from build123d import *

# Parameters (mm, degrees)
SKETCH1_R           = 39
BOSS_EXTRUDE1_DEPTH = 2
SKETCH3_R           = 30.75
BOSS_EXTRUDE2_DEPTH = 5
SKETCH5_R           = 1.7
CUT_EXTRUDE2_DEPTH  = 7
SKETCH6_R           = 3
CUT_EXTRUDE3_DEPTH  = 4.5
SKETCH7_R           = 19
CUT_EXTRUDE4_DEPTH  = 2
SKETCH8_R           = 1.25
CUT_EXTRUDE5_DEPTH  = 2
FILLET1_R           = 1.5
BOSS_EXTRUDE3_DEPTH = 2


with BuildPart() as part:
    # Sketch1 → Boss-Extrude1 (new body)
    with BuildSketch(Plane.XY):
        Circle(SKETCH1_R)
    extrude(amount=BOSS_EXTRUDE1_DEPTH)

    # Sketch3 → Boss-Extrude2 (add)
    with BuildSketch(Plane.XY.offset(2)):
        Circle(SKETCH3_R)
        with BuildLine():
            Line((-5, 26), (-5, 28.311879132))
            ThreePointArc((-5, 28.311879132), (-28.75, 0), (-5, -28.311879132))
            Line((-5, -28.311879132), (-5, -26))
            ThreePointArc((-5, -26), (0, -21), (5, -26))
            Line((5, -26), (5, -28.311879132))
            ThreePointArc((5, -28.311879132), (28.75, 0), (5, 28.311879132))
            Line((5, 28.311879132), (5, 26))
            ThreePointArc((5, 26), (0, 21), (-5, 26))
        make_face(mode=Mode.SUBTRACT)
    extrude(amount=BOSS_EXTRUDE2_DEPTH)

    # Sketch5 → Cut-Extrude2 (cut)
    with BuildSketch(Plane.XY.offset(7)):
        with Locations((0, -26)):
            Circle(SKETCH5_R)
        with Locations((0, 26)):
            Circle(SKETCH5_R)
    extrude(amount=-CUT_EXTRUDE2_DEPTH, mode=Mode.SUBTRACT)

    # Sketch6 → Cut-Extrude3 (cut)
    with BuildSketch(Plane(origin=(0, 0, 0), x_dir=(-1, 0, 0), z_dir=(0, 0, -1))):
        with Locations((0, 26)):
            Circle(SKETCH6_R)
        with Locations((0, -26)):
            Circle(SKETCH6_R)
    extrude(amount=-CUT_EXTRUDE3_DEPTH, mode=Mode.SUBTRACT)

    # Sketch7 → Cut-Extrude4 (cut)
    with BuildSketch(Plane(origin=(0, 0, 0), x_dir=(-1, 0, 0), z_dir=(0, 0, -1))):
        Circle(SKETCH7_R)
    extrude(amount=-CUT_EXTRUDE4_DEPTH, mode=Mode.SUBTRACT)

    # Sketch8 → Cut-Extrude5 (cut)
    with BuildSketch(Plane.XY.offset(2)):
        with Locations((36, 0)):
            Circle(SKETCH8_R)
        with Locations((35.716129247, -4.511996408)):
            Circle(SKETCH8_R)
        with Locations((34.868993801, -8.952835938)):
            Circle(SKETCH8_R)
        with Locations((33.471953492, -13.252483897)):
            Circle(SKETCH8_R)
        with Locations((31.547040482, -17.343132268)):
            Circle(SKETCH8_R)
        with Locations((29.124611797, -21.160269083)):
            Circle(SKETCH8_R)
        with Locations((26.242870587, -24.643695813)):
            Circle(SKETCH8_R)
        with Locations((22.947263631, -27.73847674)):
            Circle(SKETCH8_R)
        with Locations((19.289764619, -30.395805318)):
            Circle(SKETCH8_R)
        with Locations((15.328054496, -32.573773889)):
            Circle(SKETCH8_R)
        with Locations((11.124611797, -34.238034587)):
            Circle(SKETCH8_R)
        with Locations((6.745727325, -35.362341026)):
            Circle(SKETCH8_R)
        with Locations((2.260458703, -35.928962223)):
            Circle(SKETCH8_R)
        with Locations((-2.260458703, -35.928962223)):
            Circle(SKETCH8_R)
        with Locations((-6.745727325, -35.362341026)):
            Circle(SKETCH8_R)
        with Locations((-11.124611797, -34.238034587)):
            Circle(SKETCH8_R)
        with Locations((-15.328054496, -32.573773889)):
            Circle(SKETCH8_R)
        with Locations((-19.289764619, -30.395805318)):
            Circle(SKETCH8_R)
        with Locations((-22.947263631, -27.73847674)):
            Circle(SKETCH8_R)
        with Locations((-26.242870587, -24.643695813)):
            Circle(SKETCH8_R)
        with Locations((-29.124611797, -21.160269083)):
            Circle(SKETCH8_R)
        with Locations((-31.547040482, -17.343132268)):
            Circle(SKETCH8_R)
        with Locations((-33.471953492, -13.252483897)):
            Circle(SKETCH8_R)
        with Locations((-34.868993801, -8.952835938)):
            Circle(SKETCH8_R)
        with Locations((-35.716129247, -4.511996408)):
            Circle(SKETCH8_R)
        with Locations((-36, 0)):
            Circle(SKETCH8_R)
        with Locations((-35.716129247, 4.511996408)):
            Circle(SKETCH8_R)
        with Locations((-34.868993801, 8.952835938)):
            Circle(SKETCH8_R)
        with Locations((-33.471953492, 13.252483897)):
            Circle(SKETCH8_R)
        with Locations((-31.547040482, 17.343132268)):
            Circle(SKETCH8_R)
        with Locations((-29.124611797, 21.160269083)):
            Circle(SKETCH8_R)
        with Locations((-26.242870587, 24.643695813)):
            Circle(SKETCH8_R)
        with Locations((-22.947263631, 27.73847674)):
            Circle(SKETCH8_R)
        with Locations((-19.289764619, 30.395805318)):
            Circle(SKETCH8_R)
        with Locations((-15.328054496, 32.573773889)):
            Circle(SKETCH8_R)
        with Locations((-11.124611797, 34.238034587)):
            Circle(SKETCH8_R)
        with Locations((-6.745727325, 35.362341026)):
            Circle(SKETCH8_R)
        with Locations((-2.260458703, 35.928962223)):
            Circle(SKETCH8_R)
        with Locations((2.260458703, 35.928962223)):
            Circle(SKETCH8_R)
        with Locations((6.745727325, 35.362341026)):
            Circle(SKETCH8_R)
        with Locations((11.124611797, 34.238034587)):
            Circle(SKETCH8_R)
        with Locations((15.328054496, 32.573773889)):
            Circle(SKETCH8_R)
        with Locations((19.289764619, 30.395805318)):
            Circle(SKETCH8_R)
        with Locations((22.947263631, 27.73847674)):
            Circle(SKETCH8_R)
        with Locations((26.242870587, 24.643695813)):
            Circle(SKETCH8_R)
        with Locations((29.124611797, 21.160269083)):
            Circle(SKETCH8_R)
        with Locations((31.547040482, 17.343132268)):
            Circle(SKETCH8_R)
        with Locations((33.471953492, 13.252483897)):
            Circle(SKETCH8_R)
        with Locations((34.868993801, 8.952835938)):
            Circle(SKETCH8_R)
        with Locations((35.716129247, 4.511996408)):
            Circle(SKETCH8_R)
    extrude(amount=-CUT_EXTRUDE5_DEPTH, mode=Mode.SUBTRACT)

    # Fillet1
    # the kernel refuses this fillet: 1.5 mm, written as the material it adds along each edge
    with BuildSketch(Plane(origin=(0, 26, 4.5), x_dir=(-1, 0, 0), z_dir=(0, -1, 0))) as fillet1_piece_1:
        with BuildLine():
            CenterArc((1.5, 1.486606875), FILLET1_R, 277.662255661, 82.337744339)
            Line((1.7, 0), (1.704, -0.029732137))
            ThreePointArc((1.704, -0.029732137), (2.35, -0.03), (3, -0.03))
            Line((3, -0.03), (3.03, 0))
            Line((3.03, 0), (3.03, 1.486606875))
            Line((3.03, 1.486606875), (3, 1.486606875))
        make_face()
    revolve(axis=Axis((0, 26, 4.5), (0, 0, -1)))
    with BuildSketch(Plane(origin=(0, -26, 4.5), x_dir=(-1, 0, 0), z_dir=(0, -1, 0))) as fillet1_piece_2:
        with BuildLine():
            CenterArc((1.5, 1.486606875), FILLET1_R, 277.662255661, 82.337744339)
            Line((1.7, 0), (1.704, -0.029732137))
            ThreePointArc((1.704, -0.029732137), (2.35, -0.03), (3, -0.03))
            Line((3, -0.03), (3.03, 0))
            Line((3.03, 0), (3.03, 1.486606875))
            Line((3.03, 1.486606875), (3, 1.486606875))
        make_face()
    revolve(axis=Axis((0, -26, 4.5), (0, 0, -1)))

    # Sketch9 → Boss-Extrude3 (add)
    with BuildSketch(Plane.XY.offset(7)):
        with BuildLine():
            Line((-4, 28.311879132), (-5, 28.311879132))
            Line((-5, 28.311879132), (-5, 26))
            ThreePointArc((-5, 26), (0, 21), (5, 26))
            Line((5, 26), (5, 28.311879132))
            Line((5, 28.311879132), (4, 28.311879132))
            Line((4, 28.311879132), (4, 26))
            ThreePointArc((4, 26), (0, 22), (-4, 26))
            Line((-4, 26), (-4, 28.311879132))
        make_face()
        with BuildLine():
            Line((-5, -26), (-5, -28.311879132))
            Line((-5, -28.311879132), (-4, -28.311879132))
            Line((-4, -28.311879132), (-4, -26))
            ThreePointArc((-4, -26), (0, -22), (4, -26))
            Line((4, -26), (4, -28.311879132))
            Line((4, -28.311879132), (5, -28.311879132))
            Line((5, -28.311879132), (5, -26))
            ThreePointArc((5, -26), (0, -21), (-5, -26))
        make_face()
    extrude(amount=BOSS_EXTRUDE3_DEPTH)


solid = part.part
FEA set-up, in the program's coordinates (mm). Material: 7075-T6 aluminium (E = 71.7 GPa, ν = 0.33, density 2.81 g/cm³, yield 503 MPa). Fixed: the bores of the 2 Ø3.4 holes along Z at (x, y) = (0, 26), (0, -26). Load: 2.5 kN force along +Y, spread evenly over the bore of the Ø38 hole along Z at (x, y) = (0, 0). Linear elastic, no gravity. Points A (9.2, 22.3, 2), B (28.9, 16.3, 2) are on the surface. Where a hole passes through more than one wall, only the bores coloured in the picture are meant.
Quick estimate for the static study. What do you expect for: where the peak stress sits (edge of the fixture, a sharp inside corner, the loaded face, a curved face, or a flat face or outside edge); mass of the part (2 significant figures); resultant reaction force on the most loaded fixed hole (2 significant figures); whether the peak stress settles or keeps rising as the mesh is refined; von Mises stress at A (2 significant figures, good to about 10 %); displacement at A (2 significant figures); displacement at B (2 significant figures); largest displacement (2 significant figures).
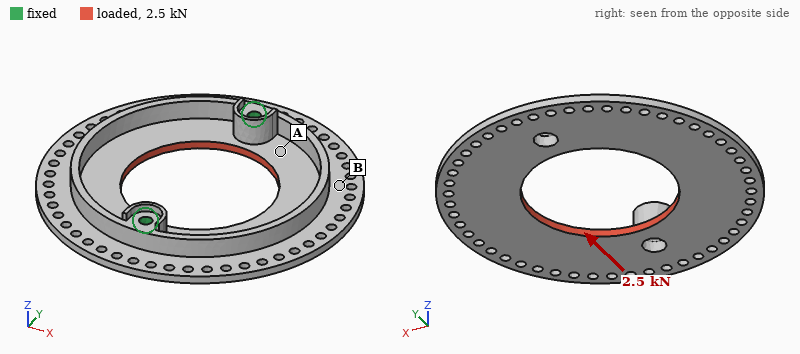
edge of the fixture
26 g
1.3 kN
keeps rising
42 MPa
21 µm
28 µm
42 µm
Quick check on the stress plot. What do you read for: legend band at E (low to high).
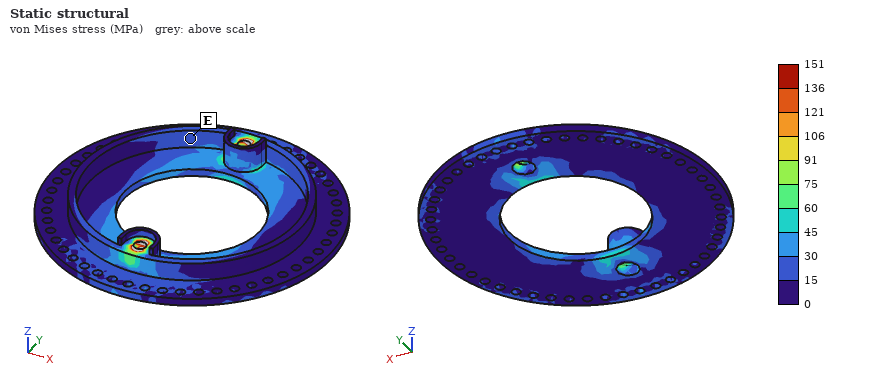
15 to 30 MPa
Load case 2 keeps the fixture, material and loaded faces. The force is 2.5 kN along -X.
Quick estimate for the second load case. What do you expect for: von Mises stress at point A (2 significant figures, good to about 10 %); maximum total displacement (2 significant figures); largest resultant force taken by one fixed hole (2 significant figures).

24 MPa
0.18 mm
1.3 kN
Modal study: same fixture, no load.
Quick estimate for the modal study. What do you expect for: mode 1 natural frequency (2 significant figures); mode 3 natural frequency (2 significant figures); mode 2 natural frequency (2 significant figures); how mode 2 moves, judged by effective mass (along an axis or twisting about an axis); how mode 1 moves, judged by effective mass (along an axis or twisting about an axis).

1900 Hz
4300 Hz
2500 Hz
along Z
twisting about Y
